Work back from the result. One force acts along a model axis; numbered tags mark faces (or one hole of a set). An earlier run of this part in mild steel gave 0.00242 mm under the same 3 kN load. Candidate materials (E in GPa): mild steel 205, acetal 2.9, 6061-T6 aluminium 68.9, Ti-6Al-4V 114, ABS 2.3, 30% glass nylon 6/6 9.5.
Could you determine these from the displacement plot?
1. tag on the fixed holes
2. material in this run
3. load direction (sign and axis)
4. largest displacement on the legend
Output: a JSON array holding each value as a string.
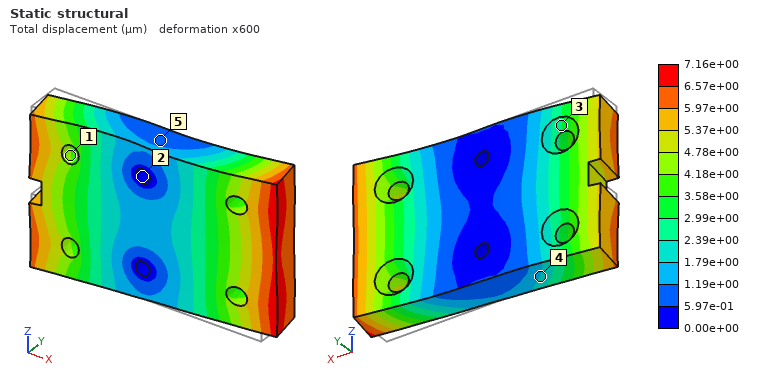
["2", "6061-T6 aluminium", "+X", "7.16e+00 µm"]
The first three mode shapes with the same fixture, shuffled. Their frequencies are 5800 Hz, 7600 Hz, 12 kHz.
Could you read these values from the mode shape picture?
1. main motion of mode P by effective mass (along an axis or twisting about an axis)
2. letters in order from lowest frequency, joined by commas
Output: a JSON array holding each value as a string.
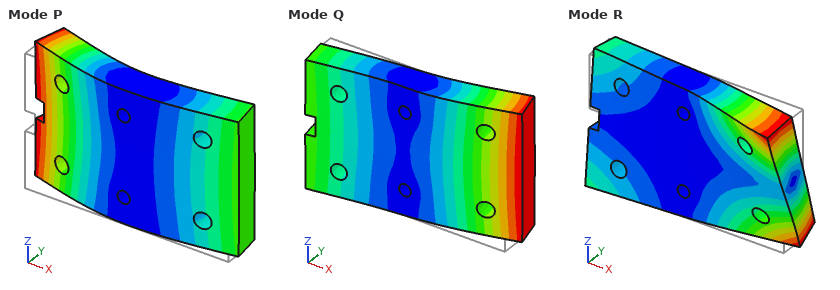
["along Y", "Q, P, R"]
